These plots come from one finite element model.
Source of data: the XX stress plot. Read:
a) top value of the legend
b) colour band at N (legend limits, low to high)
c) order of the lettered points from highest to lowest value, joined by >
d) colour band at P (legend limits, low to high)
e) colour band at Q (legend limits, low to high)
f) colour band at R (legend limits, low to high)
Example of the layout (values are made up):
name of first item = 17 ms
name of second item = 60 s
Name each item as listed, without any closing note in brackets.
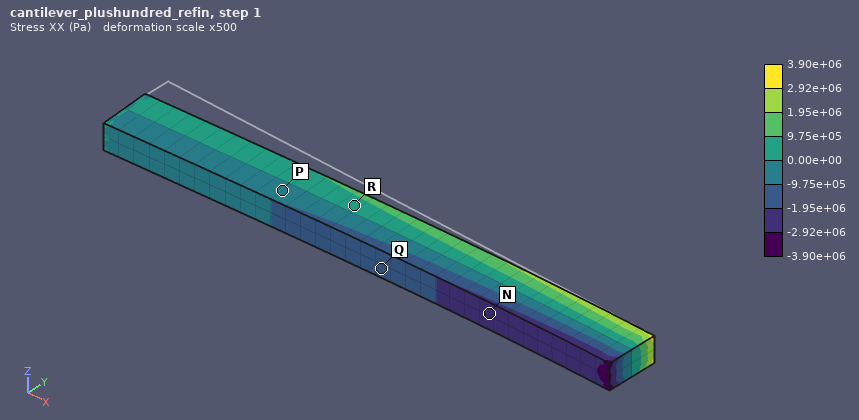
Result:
top value of the legend = 3.90e+06 Pa
colour band at N = -2.92e+06 to -1.95e+06 Pa
order of the lettered points from highest to lowest value, joined by > = R > P > Q > N
colour band at P = -9.75e+05 to 0.00e+00 Pa
colour band at Q = -1.95e+06 to -9.75e+05 Pa
colour band at R = 0.00e+00 to 9.75e+05 Pa
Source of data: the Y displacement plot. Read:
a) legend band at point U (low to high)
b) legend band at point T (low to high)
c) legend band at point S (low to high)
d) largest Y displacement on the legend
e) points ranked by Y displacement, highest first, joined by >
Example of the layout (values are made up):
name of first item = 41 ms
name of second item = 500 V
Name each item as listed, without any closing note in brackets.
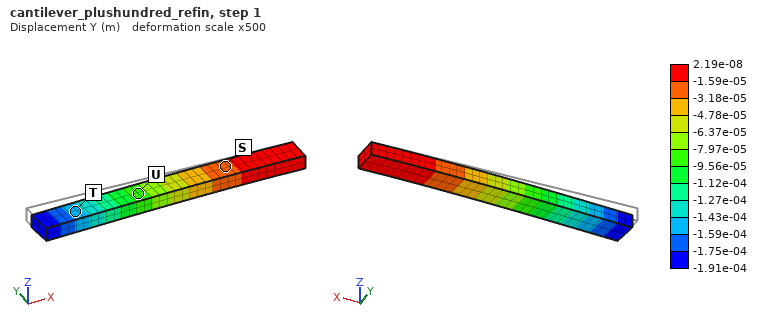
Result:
legend band at point U = -9.56e-05 to -7.97e-05 m
legend band at point T = -1.59e-04 to -1.43e-04 m
legend band at point S = -3.18e-05 to -1.59e-05 m
largest Y displacement on the legend = 2.19e-08 m
points ranked by Y displacement, highest first, joined by > = S > U > T
